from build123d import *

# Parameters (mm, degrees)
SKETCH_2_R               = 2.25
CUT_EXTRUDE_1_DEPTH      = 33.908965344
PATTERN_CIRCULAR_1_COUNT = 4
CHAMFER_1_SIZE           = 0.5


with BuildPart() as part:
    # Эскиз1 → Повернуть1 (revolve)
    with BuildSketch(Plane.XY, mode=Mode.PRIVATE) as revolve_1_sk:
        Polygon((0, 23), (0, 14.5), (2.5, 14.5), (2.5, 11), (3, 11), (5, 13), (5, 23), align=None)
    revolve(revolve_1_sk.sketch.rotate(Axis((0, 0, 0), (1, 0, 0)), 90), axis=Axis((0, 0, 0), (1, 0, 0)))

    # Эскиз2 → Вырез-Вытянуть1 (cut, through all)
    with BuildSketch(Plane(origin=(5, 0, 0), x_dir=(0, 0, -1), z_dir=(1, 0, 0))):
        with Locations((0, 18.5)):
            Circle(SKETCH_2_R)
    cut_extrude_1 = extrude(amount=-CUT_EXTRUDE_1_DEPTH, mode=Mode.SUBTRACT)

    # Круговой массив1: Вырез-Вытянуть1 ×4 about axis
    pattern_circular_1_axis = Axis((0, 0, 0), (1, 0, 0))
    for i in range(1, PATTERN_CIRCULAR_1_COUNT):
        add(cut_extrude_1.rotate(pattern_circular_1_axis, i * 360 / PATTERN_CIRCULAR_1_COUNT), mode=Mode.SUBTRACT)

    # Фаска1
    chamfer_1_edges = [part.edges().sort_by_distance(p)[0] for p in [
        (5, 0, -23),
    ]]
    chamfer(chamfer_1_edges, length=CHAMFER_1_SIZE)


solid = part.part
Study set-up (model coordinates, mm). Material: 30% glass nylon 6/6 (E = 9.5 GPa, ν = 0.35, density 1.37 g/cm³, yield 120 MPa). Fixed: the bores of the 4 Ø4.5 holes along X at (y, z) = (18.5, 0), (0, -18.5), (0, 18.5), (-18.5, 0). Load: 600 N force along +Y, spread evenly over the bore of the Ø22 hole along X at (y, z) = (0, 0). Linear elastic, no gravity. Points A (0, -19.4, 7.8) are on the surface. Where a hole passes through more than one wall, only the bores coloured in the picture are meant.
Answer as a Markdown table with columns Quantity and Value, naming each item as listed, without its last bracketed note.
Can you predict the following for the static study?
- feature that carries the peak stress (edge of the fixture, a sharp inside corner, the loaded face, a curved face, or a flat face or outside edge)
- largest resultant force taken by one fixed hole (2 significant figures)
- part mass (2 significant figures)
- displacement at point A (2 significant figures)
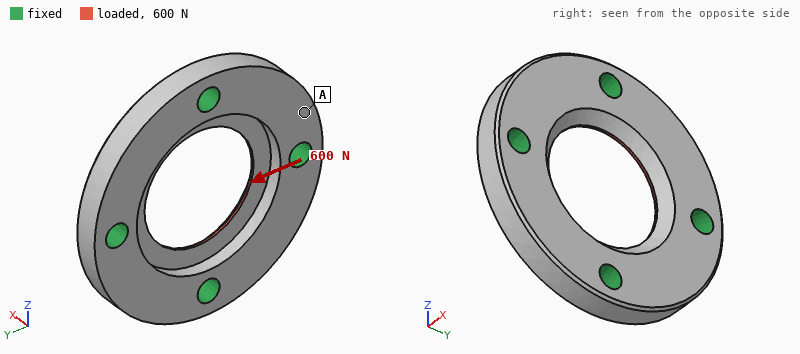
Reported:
| Quantity | Value |
|---|---|
| feature that carries the peak stress | the loaded face |
| largest resultant force taken by one fixed hole | 160 N |
| part mass | 7.2 g |
| displacement at point A | 2.0 µm |
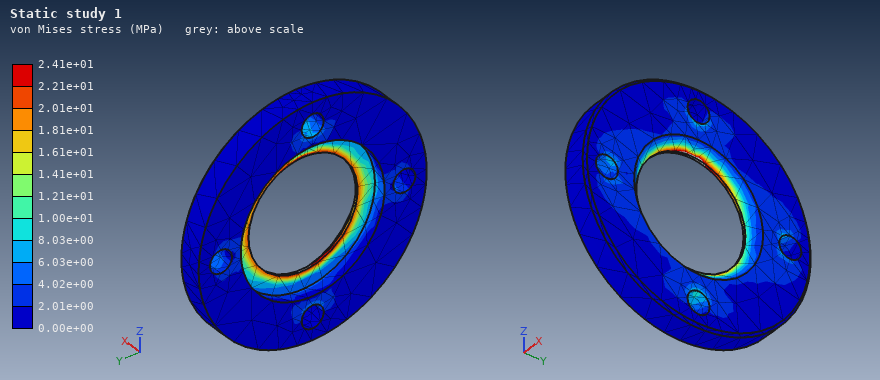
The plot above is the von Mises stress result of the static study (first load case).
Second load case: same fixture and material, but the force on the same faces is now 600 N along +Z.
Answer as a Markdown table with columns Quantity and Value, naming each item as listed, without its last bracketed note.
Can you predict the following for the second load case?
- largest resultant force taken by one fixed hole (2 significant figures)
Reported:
| Quantity | Value |
|---|---|
| largest resultant force taken by one fixed hole | 160 N |
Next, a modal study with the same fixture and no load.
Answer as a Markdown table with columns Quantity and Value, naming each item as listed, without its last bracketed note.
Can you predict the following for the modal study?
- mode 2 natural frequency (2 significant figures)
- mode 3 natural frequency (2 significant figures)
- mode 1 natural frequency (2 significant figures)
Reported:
| Quantity | Value |
|---|---|
| mode 2 natural frequency | 14 kHz |
| mode 3 natural frequency | 14 kHz |
| mode 1 natural frequency | 14 kHz |
